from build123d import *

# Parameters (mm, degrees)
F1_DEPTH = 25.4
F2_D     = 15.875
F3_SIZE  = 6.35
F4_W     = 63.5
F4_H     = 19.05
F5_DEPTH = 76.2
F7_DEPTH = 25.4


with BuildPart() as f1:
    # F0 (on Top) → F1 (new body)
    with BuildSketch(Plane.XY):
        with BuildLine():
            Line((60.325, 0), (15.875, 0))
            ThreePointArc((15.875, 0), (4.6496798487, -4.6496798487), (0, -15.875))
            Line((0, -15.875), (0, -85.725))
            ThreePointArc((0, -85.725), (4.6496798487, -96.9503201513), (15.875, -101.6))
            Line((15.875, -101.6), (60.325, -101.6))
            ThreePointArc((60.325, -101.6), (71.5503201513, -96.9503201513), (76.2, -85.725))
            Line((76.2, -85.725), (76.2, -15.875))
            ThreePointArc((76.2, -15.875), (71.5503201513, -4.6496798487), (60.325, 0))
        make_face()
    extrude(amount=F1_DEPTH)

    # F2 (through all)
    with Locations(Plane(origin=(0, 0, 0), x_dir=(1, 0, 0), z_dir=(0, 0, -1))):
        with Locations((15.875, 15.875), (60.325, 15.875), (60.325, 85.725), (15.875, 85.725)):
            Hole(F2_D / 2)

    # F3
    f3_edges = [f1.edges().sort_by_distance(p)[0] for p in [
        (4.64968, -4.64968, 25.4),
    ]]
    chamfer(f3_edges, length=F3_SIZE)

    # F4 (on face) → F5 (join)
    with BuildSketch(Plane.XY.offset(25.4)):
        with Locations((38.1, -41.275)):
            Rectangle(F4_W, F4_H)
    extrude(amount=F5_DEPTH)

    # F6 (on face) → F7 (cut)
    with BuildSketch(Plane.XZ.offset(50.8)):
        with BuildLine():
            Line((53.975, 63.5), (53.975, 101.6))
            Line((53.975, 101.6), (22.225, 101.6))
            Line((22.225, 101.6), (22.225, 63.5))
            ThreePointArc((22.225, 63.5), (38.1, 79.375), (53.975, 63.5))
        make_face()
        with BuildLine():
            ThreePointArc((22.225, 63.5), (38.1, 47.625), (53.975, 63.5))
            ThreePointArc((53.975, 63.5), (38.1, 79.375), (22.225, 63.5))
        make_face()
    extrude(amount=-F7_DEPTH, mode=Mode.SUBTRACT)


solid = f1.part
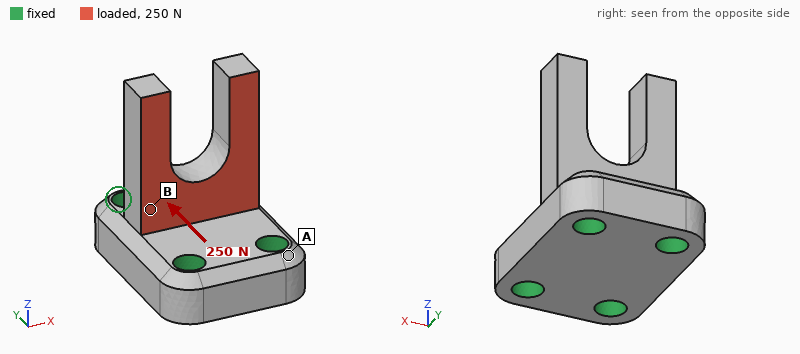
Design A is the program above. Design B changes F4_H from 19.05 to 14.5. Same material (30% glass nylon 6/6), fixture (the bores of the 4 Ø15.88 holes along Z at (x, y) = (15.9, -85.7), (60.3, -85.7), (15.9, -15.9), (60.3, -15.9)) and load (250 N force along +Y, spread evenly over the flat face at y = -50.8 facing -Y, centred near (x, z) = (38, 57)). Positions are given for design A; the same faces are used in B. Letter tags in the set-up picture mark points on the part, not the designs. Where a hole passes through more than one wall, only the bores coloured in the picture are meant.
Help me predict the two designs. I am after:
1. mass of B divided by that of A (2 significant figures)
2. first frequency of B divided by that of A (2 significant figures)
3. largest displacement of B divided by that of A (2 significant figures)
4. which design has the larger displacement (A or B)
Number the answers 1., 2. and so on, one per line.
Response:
1. 0.93
2. 0.80
3. 2.0
4. B
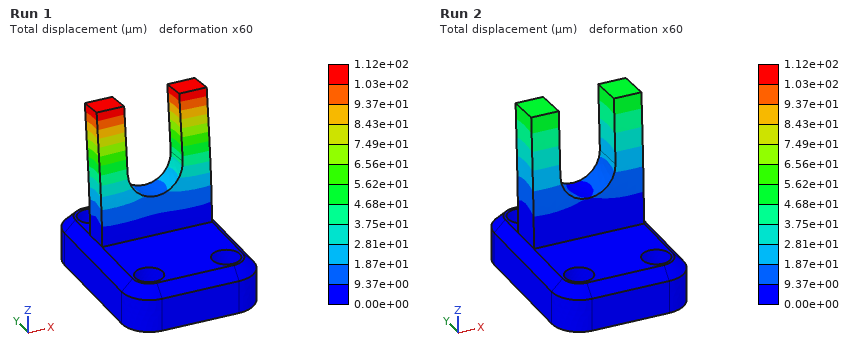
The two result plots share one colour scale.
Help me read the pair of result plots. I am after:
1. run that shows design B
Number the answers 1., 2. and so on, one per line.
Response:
1. Run 1
